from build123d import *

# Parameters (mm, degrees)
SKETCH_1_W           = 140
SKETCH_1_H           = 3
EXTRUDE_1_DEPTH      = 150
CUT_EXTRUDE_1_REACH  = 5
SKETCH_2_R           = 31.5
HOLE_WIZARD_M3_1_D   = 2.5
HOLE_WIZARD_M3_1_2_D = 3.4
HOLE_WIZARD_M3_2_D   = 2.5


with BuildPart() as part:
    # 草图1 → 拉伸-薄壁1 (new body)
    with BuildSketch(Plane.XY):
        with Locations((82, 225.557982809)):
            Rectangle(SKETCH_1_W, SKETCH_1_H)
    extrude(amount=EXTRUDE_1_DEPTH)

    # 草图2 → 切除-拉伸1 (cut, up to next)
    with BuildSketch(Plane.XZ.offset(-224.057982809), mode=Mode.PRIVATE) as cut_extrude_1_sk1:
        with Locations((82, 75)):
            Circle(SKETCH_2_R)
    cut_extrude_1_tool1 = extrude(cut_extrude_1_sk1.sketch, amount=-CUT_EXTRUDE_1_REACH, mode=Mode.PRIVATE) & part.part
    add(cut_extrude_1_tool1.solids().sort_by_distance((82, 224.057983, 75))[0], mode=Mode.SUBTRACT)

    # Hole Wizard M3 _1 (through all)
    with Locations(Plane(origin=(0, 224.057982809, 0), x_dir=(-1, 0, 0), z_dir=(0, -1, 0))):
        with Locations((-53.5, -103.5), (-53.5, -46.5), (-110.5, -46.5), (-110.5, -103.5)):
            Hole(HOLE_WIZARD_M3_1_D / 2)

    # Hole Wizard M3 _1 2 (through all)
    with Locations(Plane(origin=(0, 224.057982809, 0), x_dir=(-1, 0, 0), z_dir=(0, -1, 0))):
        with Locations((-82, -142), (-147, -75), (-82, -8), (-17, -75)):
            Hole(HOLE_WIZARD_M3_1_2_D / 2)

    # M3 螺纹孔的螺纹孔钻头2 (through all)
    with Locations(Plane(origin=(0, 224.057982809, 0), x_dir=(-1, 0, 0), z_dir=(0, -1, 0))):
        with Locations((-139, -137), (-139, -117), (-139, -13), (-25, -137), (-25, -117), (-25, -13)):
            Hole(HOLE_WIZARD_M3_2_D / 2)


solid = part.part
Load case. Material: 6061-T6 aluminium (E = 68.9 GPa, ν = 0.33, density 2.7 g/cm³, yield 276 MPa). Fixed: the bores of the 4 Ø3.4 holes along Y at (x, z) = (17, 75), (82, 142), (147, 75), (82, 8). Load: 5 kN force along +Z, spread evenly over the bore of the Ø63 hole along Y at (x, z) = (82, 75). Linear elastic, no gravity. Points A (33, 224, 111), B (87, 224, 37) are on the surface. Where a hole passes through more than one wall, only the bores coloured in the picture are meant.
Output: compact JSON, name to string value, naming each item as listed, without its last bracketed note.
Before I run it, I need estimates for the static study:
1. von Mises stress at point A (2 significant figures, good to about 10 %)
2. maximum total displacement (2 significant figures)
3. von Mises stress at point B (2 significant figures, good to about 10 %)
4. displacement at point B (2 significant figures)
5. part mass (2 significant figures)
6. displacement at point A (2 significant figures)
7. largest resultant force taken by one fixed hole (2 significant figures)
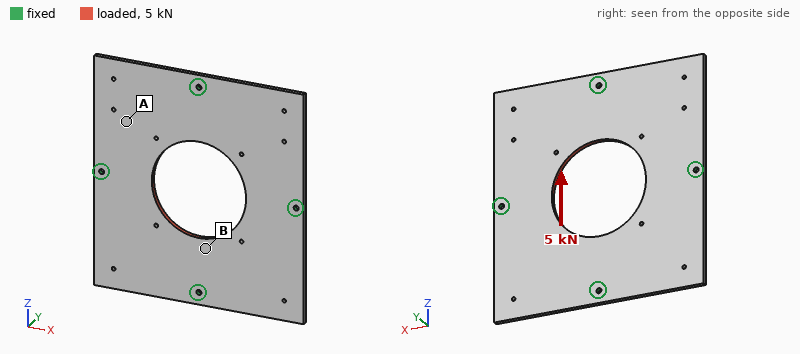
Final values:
{"von Mises stress at point A": "5.8 MPa", "maximum total displacement": "13 µm", "von Mises stress at point B": "12 MPa", "displacement at point B": "8.3 µm", "part mass": "140 g", "displacement at point A": "8.3 µm", "largest resultant force taken by one fixed hole": "1.3 kN"}
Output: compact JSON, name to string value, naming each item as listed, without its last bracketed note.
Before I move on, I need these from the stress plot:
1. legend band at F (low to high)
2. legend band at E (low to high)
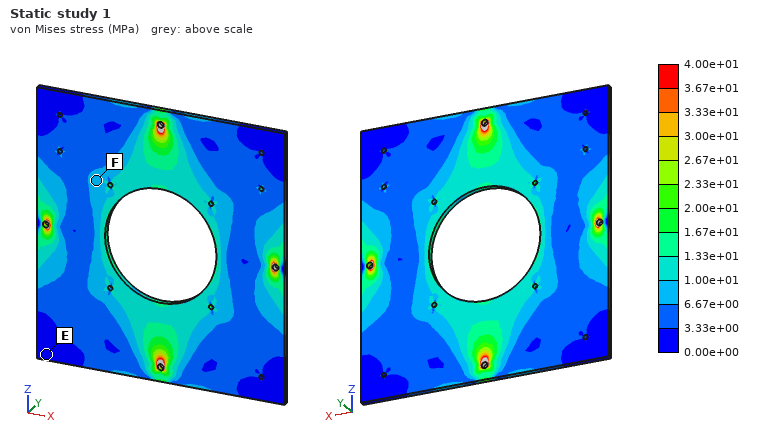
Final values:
{"legend band at F": "6.67e+00 to 1.00e+01 MPa", "legend band at E": "0.00e+00 to 3.33e+00 MPa"}
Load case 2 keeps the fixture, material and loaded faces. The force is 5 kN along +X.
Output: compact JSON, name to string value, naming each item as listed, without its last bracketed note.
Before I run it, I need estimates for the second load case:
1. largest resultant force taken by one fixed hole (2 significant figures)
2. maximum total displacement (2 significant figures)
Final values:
{"largest resultant force taken by one fixed hole": "1.3 kN", "maximum total displacement": "13 µm"}
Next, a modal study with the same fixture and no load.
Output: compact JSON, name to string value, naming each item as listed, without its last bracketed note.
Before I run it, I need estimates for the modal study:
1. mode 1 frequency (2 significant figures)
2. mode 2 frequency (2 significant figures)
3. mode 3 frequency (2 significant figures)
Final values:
{"mode 1 frequency": "810 Hz", "mode 2 frequency": "880 Hz", "mode 3 frequency": "890 Hz"}
